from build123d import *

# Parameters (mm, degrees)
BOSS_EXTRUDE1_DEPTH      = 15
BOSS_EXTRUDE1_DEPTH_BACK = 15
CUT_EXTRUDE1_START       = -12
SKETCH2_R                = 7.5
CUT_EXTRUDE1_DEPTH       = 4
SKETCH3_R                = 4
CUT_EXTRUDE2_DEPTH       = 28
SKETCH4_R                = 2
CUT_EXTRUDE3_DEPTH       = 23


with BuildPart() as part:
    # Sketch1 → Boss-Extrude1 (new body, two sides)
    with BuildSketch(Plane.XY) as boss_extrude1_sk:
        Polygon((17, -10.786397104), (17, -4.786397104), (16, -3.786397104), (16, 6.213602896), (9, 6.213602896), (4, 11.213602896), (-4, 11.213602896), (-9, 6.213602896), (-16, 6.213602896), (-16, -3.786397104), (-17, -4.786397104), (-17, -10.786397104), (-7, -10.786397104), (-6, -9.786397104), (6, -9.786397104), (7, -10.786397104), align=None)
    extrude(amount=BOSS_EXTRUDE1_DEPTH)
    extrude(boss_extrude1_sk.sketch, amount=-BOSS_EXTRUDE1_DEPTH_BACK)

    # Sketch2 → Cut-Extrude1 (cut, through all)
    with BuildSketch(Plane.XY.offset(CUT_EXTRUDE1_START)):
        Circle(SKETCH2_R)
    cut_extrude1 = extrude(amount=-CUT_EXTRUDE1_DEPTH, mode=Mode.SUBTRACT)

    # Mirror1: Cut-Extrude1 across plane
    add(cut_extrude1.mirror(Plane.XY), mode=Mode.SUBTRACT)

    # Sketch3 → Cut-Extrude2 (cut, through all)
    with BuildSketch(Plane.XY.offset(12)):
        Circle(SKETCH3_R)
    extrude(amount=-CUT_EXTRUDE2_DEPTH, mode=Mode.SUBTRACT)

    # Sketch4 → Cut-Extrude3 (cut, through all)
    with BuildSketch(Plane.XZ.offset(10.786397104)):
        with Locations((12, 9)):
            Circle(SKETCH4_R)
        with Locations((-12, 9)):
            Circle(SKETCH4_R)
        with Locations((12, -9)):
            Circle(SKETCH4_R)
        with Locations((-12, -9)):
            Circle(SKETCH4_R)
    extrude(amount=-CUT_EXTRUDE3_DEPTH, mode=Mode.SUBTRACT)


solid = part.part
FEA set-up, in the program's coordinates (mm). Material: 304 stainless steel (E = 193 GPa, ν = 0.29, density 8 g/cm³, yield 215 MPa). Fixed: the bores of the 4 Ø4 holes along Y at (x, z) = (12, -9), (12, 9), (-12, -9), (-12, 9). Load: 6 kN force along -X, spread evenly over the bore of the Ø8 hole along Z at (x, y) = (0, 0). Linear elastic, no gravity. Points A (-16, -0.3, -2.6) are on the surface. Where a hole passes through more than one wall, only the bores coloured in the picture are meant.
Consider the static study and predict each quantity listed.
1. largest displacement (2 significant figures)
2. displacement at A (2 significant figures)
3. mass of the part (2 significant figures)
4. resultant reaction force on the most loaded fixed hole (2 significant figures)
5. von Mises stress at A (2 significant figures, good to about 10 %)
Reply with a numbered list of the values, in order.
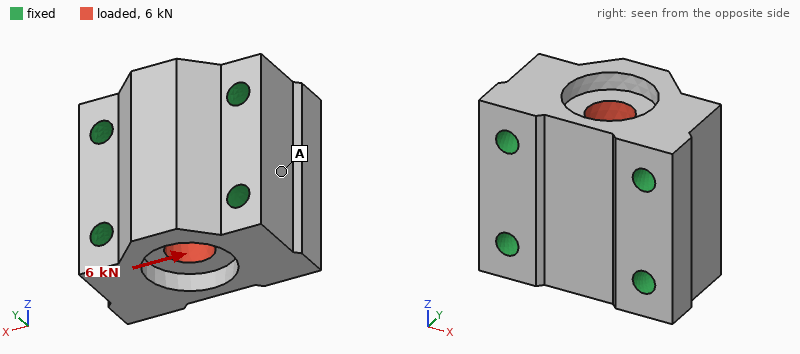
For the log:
1. 0.72 µm
2. 0.27 µm
3. 120 g
4. 1.5 kN
5. 4.1 MPa
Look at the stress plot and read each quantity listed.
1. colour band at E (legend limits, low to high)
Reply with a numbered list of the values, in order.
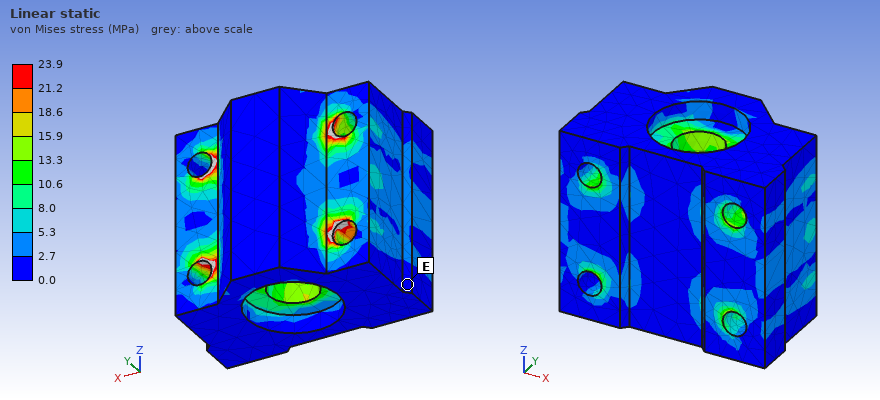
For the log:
1. 0.0 to 2.7 MPa
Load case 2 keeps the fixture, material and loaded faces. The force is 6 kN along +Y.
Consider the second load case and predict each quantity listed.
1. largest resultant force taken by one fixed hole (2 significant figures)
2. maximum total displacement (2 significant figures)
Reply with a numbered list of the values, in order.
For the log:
1. 1.5 kN
2. 1.3 µm
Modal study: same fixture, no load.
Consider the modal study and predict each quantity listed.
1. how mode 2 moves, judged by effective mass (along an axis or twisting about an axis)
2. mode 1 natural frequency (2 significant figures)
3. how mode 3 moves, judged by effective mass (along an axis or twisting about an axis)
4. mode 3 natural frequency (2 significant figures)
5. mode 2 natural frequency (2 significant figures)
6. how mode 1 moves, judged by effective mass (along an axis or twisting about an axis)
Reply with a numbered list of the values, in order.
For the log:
1. along Y
2. 49 kHz
3. along Z
4. 66 kHz
5. 56 kHz
6. along Z
